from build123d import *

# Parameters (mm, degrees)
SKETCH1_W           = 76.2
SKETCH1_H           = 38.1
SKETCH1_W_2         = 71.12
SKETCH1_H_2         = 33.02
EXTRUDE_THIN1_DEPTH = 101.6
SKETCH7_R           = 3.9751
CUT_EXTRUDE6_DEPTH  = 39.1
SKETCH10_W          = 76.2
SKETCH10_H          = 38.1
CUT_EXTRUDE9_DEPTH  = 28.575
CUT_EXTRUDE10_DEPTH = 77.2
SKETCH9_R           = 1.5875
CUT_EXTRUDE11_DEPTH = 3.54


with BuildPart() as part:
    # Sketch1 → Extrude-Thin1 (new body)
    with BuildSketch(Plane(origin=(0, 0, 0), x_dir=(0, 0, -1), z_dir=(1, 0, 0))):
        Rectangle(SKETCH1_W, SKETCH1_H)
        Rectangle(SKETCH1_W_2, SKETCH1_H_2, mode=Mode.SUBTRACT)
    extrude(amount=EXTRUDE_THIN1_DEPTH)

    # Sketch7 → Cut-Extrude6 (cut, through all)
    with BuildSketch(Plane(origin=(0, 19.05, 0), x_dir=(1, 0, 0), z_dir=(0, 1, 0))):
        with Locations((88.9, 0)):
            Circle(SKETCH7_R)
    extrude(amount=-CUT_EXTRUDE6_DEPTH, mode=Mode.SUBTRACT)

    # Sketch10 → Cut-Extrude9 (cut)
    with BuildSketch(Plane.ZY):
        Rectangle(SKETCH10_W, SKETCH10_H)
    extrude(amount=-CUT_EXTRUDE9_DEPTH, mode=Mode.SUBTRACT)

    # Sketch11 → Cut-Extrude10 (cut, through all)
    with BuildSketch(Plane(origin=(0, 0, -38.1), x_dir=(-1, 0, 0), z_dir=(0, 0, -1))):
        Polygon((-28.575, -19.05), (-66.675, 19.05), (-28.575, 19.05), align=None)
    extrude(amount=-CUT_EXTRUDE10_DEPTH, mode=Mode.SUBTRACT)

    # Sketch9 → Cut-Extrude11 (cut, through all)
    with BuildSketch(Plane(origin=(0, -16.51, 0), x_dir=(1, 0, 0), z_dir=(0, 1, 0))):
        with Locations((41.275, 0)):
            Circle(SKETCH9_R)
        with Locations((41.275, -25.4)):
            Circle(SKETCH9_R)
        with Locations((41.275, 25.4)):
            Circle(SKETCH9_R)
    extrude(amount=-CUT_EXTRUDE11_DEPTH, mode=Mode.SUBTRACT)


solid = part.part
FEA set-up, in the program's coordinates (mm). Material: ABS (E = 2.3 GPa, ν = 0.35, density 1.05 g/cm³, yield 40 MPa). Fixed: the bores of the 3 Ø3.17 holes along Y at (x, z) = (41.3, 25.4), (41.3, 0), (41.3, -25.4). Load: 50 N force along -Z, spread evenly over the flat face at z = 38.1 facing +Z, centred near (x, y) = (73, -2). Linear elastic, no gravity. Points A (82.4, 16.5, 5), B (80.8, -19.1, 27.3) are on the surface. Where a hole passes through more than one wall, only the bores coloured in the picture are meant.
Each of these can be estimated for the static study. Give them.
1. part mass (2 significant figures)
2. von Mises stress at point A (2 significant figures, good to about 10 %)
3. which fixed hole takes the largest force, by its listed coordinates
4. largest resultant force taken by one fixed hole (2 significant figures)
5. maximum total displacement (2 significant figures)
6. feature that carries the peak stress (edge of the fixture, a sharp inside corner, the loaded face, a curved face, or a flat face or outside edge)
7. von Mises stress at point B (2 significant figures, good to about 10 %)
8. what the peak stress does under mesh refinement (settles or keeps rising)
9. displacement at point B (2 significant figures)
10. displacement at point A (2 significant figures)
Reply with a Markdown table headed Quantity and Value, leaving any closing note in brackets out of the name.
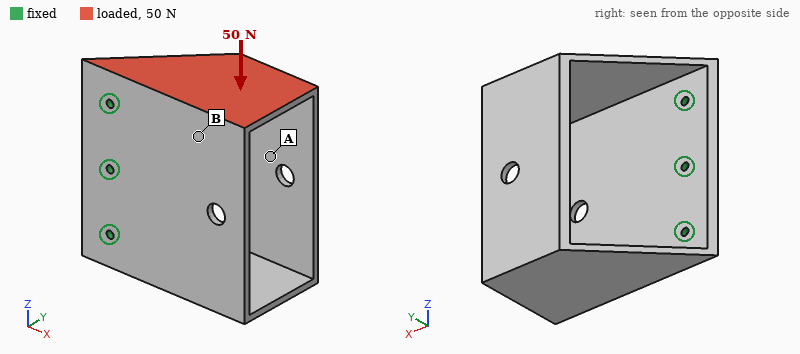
| Quantity | Value |
|---|---|
| part mass | 31 g |
| von Mises stress at point A | 1.2 MPa |
| which fixed hole takes the largest force, by its listed coordinates | (41.3, 25.4) |
| largest resultant force taken by one fixed hole | 39 N |
| maximum total displacement | 1.3 mm |
| feature that carries the peak stress | edge of the fixture |
| von Mises stress at point B | 2.7 MPa |
| what the peak stress does under mesh refinement | keeps rising |
| displacement at point B | 0.26 mm |
| displacement at point A | 1.1 mm |
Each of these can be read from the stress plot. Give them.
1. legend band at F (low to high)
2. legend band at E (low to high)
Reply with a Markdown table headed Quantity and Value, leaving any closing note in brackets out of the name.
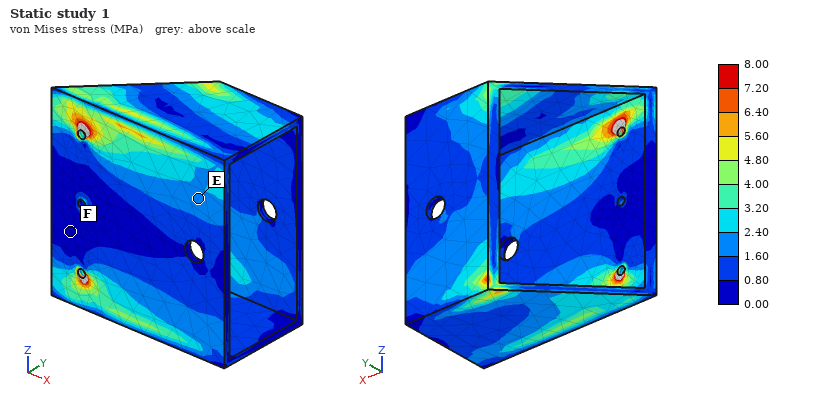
| Quantity | Value |
|---|---|
| legend band at F | 0.00 to 0.80 MPa |
| legend band at E | 1.60 to 2.40 MPa |
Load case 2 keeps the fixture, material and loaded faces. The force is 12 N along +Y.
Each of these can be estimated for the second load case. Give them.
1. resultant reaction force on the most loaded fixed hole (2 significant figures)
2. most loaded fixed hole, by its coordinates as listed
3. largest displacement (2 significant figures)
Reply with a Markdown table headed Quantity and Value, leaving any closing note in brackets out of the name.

| Quantity | Value |
|---|---|
| resultant reaction force on the most loaded fixed hole | 12 N |
| most loaded fixed hole, by its coordinates as listed | (41.3, 25.4) |
| largest displacement | 1.2 mm |
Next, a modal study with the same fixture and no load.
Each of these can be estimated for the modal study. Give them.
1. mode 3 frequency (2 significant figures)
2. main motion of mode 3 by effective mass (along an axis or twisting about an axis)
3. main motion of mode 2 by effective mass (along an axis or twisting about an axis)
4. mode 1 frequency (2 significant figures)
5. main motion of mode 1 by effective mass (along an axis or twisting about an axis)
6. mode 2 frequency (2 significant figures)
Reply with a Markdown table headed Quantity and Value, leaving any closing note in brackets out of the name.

| Quantity | Value |
|---|---|
| mode 3 frequency | 340 Hz |
| main motion of mode 3 by effective mass | along Z |
| main motion of mode 2 by effective mass | along Z |
| mode 1 frequency | 130 Hz |
| main motion of mode 1 by effective mass | along Y |
| mode 2 frequency | 190 Hz |
